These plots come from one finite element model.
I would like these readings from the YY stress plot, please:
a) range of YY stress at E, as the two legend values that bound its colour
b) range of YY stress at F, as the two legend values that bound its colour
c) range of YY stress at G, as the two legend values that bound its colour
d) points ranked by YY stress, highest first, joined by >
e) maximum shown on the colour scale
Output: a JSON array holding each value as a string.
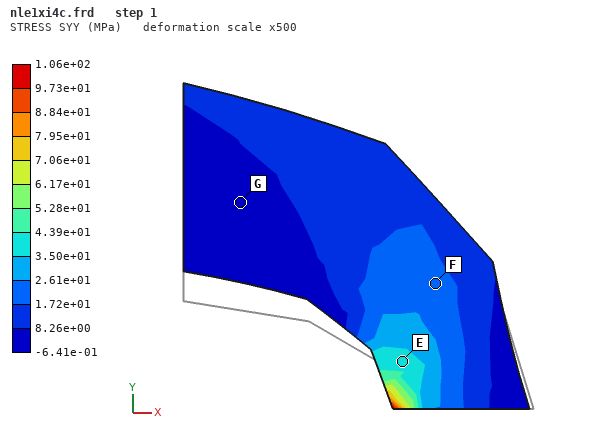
["3.50e+01 to 4.39e+01 MPa", "1.72e+01 to 2.61e+01 MPa", "-6.41e-01 to 8.26e+00 MPa", "E > F > G", "1.06e+02 MPa"]
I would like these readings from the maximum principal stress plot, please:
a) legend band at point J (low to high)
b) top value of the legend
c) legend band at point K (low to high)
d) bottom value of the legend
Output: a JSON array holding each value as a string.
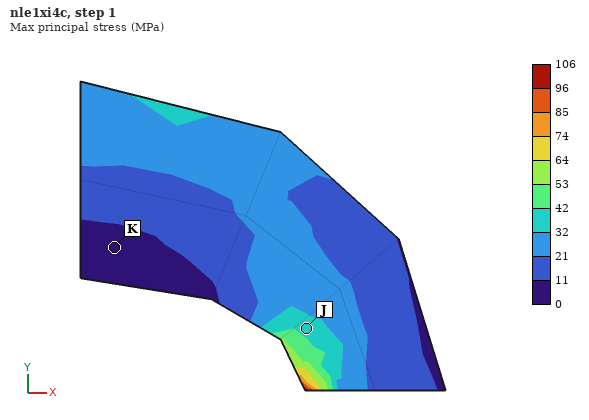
["32 to 42 MPa", "106 MPa", "0 to 11 MPa", "0 MPa"]
